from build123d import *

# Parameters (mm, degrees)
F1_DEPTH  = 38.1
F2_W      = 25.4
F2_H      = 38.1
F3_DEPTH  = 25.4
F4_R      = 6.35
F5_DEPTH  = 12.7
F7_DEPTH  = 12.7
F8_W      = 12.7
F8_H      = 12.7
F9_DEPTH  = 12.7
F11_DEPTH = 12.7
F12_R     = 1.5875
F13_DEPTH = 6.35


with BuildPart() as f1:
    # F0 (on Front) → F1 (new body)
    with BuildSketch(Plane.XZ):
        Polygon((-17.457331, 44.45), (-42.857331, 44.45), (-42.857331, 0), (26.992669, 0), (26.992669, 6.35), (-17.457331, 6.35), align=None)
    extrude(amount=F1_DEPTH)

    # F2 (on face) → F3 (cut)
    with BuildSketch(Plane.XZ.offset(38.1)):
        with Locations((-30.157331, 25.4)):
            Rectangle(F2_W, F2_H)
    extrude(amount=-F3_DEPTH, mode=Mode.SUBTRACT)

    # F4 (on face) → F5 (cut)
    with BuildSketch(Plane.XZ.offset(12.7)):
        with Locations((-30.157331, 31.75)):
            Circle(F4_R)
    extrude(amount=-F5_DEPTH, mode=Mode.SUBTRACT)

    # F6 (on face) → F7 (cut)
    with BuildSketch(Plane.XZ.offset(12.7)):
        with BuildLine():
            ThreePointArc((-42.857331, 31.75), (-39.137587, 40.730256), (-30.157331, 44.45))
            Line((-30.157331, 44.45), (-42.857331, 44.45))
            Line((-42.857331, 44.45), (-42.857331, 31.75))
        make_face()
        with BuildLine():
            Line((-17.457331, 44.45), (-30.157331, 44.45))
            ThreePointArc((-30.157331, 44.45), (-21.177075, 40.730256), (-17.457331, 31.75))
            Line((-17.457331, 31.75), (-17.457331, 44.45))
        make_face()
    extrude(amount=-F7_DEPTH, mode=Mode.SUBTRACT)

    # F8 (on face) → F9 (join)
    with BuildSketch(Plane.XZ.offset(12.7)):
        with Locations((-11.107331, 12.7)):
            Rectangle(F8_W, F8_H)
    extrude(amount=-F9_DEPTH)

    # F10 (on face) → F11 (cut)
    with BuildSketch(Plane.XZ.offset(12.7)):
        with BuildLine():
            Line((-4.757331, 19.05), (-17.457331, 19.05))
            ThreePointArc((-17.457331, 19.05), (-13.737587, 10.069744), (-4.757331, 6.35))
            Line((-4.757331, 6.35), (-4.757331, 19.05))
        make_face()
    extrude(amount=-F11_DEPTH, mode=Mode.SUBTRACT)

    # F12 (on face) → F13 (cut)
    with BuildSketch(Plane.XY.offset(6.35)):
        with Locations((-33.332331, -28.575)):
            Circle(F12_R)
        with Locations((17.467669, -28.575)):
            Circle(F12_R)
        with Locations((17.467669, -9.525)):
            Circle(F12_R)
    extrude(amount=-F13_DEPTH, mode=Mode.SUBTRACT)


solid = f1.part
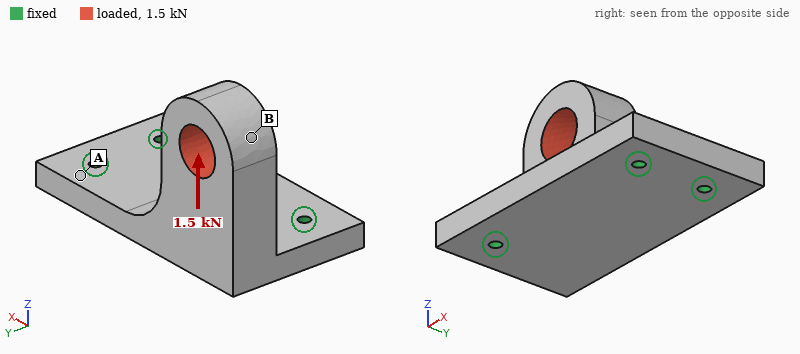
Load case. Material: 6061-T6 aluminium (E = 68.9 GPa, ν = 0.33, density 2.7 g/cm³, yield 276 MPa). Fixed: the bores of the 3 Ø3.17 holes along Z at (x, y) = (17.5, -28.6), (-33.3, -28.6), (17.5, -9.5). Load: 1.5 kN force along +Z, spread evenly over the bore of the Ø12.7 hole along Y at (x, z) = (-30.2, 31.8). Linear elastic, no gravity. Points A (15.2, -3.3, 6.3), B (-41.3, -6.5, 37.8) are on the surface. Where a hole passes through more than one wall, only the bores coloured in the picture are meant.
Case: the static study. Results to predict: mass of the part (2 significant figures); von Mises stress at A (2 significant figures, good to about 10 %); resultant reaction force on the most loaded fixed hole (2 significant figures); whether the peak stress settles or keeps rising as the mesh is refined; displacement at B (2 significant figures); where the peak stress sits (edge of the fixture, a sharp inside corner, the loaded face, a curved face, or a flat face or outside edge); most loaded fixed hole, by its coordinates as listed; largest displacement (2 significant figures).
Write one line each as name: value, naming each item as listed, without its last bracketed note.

mass of the part: 73 g
von Mises stress at A: 40 MPa
resultant reaction force on the most loaded fixed hole: 1.3 kN
whether the peak stress settles or keeps rising as the mesh is refined: keeps rising
displacement at B: 0.23 mm
where the peak stress sits: edge of the fixture
most loaded fixed hole, by its coordinates as listed: (-33.3, -28.6)
largest displacement: 0.27 mm
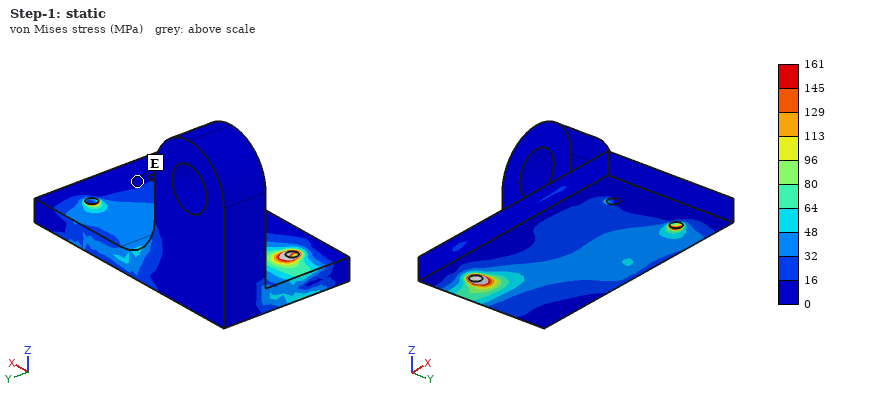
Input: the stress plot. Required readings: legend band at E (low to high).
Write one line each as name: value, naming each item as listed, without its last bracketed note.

legend band at E: 0 to 16 MPa
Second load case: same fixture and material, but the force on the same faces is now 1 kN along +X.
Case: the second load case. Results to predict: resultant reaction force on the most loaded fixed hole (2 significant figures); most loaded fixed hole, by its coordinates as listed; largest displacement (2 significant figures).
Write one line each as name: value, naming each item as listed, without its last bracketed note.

resultant reaction force on the most loaded fixed hole: 700 N
most loaded fixed hole, by its coordinates as listed: (-33.3, -28.6)
largest displacement: 0.14 mm
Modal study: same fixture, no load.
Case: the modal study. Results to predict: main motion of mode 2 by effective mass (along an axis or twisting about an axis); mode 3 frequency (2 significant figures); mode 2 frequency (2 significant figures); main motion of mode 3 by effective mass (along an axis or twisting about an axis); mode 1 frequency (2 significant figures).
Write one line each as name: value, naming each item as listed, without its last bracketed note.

main motion of mode 2 by effective mass: along X
mode 3 frequency: 6300 Hz
mode 2 frequency: 4300 Hz
main motion of mode 3 by effective mass: along Z
mode 1 frequency: 2100 Hz
